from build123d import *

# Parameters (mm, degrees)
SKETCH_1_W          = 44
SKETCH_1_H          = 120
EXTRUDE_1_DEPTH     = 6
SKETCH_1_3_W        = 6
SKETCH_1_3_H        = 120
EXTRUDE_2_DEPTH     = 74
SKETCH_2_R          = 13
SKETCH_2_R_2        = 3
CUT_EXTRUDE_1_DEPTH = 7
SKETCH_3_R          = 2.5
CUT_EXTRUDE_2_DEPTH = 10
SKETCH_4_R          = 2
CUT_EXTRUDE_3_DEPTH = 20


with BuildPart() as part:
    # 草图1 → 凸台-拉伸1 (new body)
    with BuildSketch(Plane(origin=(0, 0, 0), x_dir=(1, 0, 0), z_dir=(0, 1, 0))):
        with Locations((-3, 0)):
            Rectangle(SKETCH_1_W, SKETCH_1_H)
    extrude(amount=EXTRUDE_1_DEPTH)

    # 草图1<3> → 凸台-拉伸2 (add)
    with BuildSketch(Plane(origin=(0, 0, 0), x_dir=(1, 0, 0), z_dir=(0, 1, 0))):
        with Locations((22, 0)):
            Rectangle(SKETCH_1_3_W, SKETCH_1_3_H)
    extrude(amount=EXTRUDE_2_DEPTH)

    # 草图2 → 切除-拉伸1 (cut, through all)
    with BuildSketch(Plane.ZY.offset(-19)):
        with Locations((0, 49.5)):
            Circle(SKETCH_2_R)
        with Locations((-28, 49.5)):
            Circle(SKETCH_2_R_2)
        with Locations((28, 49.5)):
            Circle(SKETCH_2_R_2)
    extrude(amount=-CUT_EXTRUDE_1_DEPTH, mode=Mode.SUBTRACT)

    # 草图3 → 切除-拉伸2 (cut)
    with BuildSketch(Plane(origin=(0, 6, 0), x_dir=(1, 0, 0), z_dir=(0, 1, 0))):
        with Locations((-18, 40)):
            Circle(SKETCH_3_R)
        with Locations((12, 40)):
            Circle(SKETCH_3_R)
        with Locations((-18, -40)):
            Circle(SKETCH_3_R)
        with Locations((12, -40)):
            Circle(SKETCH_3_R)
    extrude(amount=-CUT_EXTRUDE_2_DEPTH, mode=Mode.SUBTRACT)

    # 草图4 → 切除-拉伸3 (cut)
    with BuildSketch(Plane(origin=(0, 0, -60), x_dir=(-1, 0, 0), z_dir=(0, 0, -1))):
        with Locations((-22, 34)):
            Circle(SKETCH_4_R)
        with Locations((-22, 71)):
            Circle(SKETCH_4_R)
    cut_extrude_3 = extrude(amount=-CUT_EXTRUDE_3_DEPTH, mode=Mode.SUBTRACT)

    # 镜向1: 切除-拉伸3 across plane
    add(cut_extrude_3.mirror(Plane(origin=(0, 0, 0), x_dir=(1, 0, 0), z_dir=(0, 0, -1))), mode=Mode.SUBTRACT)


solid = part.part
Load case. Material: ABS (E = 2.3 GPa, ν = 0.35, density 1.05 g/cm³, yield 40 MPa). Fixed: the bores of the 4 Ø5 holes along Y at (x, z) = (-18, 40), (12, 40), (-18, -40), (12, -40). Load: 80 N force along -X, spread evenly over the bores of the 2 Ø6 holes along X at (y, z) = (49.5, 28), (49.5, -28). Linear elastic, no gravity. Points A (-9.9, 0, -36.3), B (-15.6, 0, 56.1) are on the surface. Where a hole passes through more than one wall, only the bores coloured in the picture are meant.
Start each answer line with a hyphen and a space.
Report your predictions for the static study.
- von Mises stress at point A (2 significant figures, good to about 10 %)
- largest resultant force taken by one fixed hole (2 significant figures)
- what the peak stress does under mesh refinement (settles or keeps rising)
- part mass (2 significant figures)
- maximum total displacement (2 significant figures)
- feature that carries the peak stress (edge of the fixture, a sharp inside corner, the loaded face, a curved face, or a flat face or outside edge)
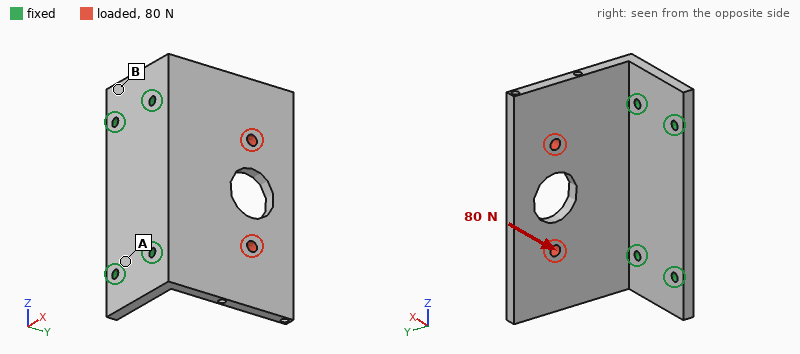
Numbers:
- 1.0 MPa
- 46 N
- keeps rising
- 84 g
- 1.5 mm
- edge of the fixture
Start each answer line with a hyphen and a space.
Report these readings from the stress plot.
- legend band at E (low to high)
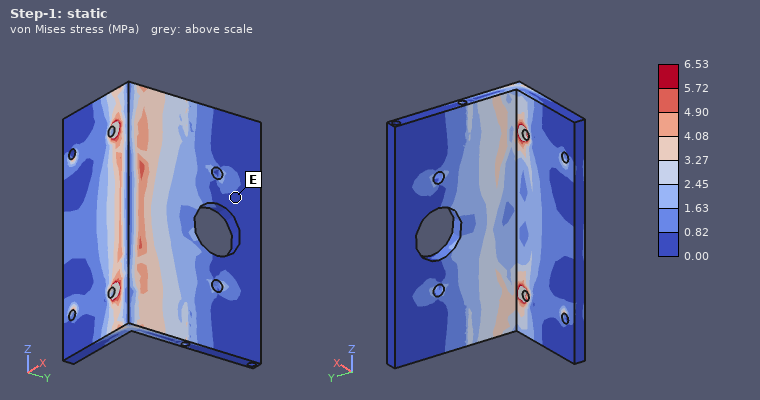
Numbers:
- 0.00 to 0.82 MPa
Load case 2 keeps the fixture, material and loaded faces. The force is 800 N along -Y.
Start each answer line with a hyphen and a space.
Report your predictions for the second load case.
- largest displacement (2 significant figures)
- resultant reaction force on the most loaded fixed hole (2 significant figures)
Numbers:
- 0.94 mm
- 460 N
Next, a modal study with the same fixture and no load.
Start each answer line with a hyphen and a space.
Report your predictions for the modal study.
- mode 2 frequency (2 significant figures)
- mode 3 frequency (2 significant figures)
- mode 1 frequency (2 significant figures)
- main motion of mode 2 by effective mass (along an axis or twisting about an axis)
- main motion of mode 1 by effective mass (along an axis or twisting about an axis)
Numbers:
- 420 Hz
- 950 Hz
- 240 Hz
- twisting about Y
- along X
